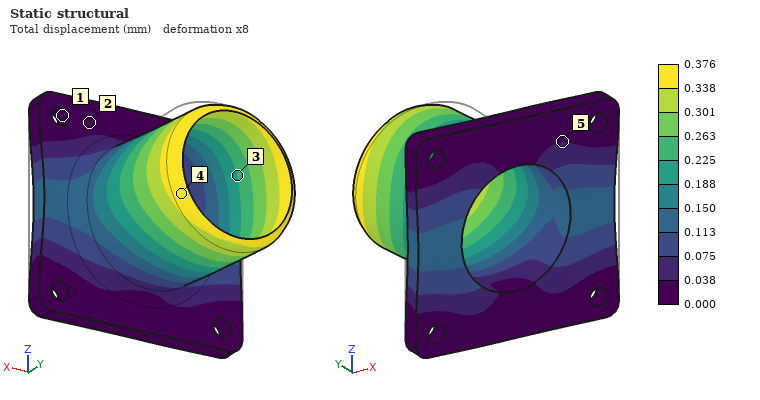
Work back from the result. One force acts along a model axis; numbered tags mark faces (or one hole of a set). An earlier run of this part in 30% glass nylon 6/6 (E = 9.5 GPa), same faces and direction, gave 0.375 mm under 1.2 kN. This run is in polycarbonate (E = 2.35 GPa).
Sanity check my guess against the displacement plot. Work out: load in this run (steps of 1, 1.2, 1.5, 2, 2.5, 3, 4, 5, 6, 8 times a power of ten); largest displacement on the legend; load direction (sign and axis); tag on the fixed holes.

300 N
0.376 mm
-X
1
